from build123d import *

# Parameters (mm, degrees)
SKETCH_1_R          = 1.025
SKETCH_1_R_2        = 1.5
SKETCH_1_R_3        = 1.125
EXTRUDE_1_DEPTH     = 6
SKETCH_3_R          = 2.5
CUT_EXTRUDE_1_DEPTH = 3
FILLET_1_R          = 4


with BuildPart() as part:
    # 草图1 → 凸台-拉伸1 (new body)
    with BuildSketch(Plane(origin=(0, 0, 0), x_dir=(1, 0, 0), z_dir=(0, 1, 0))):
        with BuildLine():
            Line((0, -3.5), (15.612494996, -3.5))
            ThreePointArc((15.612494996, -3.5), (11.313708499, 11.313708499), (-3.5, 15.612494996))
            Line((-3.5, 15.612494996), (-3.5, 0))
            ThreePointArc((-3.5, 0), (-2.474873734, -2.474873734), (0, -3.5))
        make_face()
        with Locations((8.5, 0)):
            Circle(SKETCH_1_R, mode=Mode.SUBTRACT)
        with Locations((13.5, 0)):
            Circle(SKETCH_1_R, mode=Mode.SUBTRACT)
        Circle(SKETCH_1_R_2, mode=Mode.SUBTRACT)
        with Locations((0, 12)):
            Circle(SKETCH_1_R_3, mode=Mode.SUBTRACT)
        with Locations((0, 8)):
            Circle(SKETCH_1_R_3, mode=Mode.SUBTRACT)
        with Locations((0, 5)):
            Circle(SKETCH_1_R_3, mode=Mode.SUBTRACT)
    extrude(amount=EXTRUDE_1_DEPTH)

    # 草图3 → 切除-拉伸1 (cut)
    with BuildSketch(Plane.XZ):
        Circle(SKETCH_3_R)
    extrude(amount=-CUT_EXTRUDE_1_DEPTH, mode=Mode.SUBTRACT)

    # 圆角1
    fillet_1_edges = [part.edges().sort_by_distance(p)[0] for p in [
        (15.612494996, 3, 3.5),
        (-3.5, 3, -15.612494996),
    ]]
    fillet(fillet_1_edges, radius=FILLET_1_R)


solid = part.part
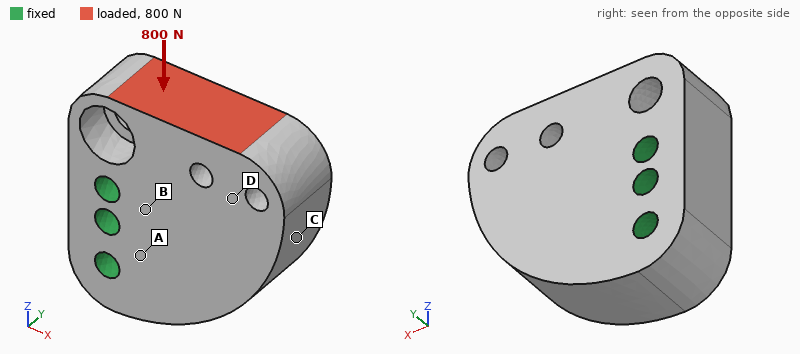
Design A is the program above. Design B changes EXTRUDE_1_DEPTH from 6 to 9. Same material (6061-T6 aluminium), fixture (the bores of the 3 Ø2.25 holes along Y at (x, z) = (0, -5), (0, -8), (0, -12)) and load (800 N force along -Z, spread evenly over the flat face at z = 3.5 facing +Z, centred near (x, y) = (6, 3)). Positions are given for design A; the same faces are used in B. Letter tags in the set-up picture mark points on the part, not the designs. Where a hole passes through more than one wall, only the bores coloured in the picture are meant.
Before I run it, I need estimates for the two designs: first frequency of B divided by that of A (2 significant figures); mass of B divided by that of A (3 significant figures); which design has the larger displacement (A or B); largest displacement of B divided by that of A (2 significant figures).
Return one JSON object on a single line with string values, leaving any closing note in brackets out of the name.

{"first frequency of B divided by that of A": "1.3", "mass of B divided by that of A": "1.51", "which design has the larger displacement": "A", "largest displacement of B divided by that of A": "0.66"}
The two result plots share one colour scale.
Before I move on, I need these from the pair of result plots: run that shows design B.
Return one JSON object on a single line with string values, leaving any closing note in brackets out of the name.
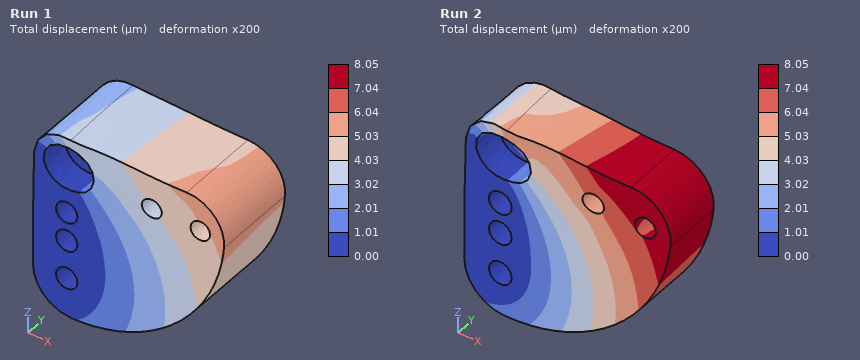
{"run that shows design B": "Run 1"}
